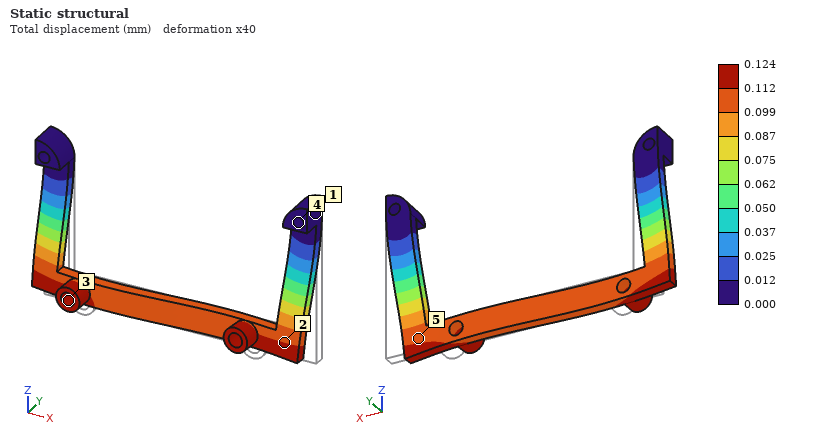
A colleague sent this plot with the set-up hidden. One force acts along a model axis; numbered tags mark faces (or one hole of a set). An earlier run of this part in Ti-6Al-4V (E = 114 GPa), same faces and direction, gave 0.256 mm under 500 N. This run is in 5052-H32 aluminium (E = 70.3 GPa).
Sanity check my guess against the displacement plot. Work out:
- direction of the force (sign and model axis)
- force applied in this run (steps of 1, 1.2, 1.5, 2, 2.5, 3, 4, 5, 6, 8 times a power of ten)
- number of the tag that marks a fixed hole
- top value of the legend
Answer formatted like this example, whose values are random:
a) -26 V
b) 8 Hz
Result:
a) -X
b) 150 N
c) 4
d) 0.124 mm
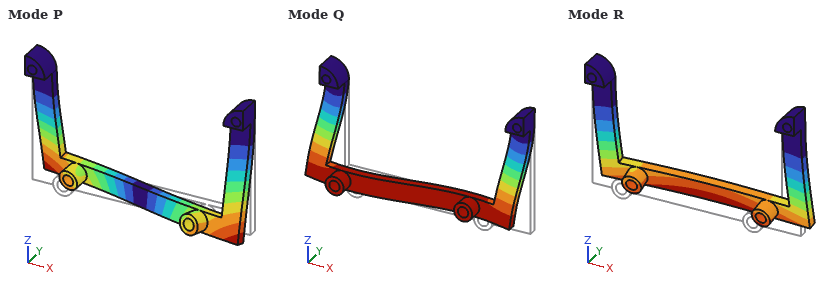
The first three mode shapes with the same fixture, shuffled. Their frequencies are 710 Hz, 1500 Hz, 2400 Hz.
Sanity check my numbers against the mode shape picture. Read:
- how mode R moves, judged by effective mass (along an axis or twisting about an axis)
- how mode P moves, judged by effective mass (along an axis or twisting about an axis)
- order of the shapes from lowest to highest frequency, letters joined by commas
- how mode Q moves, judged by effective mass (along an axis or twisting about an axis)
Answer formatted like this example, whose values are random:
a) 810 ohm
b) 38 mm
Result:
a) along Y
b) twisting about Z
c) R, P, Q
d) along X
